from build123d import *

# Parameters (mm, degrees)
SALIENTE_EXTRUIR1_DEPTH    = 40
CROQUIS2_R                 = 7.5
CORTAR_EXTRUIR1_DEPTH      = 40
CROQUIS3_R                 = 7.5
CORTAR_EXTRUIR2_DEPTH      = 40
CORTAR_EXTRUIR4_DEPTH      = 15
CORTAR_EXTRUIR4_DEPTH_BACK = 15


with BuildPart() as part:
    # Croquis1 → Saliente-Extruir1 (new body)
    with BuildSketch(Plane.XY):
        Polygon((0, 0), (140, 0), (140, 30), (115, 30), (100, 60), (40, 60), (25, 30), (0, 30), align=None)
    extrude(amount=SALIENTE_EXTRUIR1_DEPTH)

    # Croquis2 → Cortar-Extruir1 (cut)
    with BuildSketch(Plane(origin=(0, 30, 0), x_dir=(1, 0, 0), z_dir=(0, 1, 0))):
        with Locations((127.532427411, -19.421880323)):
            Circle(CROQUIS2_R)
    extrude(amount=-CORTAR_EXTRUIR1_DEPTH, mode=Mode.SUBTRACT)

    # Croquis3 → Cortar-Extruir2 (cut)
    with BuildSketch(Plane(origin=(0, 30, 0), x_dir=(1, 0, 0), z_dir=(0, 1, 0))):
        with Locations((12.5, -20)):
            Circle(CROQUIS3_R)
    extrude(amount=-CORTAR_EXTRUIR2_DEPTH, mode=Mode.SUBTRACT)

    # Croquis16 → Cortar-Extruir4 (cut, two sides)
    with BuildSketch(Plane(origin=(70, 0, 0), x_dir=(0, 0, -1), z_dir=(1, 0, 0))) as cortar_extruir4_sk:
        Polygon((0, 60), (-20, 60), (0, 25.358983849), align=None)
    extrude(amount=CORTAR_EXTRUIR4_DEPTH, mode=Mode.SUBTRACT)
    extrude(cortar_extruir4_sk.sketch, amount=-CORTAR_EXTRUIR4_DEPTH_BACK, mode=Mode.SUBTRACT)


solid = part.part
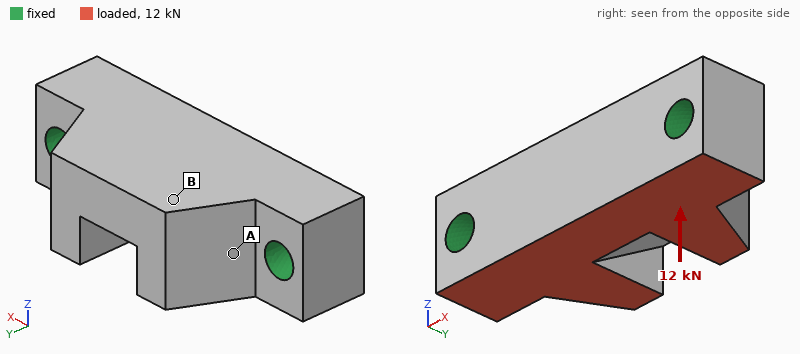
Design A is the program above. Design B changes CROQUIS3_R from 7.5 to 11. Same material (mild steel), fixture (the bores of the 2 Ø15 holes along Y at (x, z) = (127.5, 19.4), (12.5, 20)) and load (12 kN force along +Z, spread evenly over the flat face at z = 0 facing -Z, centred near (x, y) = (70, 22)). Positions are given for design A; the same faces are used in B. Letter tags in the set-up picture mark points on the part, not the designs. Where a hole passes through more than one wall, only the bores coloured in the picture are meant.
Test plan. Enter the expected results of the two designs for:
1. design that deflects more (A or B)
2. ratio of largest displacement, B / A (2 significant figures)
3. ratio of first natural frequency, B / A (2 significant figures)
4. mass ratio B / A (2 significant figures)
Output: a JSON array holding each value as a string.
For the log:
["A", "0.87", "1.1", "0.97"]
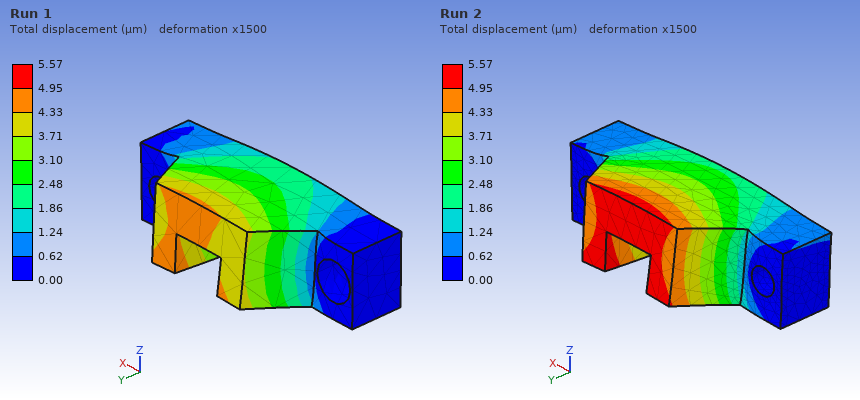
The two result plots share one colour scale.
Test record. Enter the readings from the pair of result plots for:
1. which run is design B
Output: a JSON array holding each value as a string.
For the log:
["Run 1"]
